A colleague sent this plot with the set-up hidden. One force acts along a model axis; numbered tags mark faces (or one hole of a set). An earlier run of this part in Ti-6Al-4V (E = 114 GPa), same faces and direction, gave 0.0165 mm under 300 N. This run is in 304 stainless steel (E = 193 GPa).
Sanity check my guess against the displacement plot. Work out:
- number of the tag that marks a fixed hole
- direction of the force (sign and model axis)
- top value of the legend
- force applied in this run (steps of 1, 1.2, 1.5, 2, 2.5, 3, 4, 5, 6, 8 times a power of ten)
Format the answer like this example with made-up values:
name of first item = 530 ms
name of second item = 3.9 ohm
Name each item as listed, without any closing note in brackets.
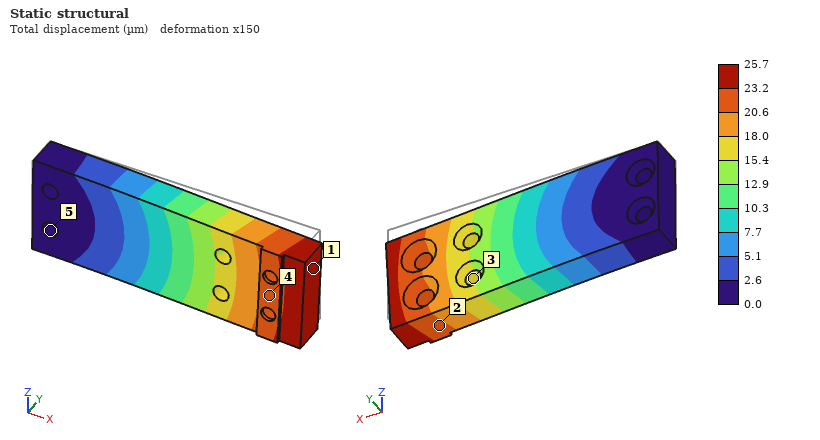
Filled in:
number of the tag that marks a fixed hole = 5
direction of the force = -Z
top value of the legend = 25.7 µm
force applied in this run = 800 N
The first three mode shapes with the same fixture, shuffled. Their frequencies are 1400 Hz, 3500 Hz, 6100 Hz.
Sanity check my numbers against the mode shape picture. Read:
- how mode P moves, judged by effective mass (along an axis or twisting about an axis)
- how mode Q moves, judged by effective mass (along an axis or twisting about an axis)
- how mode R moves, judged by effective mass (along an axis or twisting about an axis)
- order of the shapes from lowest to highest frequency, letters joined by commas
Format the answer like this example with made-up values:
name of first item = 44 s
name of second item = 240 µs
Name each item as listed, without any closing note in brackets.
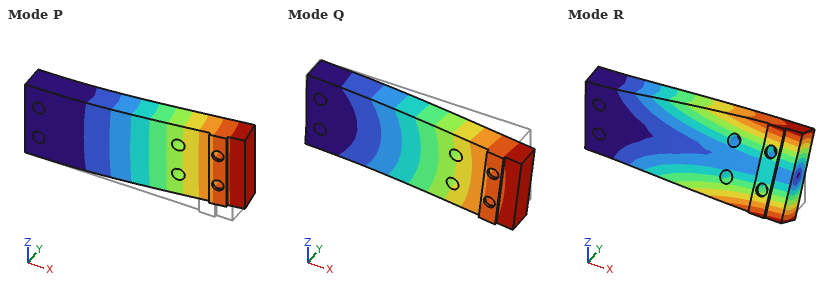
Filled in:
how mode P moves, judged by effective mass = along Y
how mode Q moves, judged by effective mass = along Z
how mode R moves, judged by effective mass = twisting about X
order of the shapes from lowest to highest frequency, letters joined by commas = P, Q, R
